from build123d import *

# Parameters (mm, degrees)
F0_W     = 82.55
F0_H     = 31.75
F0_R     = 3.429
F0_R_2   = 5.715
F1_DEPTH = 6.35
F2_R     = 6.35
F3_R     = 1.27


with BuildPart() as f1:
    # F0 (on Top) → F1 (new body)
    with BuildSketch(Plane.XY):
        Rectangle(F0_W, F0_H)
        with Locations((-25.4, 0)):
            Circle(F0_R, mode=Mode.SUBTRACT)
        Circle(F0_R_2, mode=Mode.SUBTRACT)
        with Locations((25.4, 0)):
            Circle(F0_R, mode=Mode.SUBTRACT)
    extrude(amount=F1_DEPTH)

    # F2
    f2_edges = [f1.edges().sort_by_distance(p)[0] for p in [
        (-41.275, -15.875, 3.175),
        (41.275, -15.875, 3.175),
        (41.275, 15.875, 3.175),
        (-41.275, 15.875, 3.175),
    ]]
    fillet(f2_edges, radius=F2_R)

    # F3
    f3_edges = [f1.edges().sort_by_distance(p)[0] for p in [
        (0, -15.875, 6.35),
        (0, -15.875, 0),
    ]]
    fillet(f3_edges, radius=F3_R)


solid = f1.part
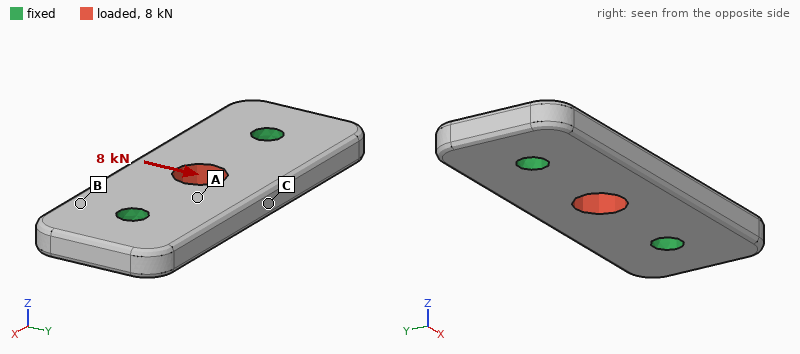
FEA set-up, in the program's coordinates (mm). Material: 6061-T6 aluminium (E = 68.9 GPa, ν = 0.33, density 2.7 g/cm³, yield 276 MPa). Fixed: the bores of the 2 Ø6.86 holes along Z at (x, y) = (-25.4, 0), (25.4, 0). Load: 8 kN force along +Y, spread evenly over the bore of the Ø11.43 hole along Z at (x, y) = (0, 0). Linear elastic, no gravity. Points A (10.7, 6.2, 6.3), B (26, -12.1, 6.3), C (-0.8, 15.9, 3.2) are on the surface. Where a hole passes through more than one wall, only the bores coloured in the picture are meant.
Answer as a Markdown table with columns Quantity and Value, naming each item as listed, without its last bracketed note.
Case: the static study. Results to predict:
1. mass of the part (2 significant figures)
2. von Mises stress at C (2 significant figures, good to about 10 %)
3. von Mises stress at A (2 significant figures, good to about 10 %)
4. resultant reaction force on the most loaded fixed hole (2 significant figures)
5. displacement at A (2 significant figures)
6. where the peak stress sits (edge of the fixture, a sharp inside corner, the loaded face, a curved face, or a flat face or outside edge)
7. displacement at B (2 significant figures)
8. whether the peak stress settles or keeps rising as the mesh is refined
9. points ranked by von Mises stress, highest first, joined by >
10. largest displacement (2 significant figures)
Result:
| Quantity | Value |
|---|---|
| mass of the part | 41 g |
| von Mises stress at C | 84 MPa |
| von Mises stress at A | 45 MPa |
| resultant reaction force on the most loaded fixed hole | 4.0 kN |
| displacement at A | 21 µm |
| where the peak stress sits | edge of the fixture |
| displacement at B | 8.1 µm |
| whether the peak stress settles or keeps rising as the mesh is refined | keeps rising |
| points ranked by von Mises stress, highest first, joined by > | C > A > B |
| largest displacement | 33 µm |
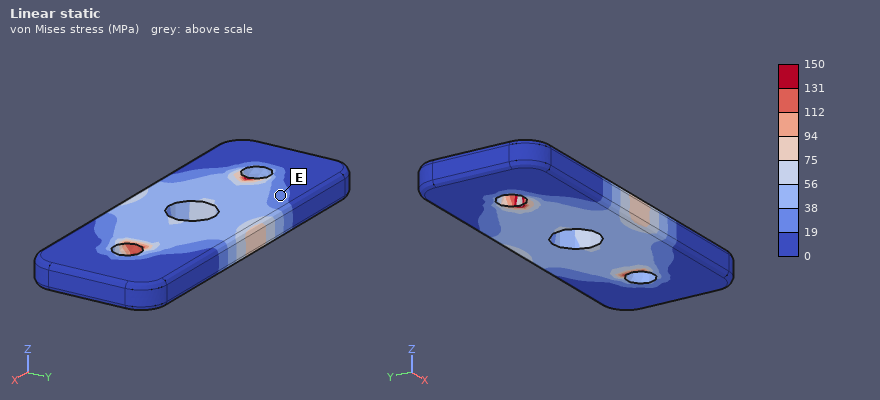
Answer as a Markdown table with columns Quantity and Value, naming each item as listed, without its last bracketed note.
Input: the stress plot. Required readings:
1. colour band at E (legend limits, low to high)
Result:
| Quantity | Value |
|---|---|
| colour band at E | 19 to 38 MPa |
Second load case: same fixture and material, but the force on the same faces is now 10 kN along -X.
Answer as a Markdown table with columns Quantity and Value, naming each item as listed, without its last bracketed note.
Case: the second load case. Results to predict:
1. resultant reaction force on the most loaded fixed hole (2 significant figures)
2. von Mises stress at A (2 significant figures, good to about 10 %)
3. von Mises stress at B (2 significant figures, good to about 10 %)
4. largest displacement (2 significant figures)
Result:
| Quantity | Value |
|---|---|
| resultant reaction force on the most loaded fixed hole | 5.0 kN |
| von Mises stress at A | 36 MPa |
| von Mises stress at B | 10 MPa |
| largest displacement | 14 µm |
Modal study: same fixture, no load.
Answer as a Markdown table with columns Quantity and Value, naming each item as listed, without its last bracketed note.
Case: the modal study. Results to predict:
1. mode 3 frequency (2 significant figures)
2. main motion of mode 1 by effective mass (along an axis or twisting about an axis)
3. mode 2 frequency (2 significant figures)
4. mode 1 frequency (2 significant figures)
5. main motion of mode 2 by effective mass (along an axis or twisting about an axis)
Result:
| Quantity | Value |
|---|---|
| mode 3 frequency | 18 kHz |
| main motion of mode 1 by effective mass | along Z |
| mode 2 frequency | 12 kHz |
| mode 1 frequency | 11 kHz |
| main motion of mode 2 by effective mass | twisting about X |
